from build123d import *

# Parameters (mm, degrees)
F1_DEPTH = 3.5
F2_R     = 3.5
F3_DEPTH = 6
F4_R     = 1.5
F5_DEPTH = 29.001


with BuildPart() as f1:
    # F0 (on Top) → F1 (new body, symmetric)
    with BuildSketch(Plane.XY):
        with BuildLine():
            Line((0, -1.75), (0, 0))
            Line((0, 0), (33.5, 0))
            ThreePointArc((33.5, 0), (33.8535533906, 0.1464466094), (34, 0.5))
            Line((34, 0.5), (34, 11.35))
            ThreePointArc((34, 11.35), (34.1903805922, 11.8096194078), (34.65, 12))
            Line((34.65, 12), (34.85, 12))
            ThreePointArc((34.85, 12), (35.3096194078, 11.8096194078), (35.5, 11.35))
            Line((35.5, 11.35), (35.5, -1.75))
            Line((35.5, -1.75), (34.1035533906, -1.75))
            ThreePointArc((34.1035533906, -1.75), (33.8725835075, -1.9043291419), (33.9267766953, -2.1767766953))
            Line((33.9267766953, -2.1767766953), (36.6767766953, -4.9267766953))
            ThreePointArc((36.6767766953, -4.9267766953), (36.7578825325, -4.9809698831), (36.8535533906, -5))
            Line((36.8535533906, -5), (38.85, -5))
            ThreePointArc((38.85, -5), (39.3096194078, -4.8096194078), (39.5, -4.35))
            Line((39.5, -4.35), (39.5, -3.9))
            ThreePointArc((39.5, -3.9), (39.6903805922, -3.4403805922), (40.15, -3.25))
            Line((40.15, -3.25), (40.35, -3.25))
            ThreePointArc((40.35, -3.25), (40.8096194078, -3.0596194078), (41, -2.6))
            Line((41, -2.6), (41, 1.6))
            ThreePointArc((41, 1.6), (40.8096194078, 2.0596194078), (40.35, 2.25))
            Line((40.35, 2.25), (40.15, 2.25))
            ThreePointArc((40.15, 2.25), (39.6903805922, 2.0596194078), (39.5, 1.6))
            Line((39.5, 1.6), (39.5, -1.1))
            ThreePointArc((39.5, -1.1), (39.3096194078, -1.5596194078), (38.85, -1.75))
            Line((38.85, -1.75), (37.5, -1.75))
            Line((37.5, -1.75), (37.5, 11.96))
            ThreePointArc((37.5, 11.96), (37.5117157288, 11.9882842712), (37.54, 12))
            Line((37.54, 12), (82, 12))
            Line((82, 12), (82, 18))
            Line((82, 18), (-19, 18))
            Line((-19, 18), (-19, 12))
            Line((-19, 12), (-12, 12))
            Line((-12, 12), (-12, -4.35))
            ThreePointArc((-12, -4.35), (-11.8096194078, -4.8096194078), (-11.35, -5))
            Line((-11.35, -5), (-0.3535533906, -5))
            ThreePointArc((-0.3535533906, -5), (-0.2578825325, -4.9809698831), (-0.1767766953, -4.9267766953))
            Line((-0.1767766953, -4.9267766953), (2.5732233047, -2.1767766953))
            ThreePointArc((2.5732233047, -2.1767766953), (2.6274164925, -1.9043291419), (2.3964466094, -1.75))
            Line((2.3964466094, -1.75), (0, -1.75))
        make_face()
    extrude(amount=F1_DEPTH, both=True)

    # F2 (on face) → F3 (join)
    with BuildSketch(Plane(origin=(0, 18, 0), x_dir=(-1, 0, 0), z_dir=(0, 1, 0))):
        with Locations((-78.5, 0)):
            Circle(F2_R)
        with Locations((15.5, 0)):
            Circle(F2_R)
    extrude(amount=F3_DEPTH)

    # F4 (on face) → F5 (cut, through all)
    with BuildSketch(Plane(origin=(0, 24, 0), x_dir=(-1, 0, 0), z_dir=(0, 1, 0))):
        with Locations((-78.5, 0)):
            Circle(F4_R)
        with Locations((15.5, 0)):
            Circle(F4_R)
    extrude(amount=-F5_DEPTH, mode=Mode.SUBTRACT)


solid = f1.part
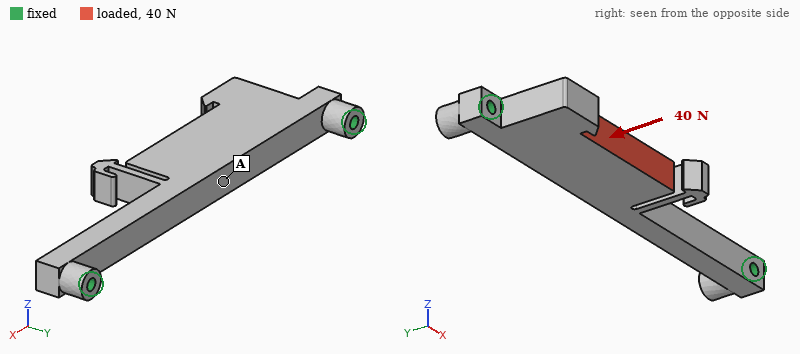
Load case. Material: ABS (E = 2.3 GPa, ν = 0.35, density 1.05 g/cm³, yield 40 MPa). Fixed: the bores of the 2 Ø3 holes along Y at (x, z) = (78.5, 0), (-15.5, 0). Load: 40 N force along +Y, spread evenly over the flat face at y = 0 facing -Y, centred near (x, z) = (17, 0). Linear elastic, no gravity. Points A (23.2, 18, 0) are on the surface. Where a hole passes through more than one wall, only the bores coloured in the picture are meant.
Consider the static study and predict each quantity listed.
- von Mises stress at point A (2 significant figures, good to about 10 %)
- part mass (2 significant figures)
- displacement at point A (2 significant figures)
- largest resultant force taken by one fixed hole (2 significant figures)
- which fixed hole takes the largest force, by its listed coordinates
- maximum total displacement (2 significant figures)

1.1 MPa
9.7 g
0.20 mm
29 N
(-15.5, 0)
0.27 mm
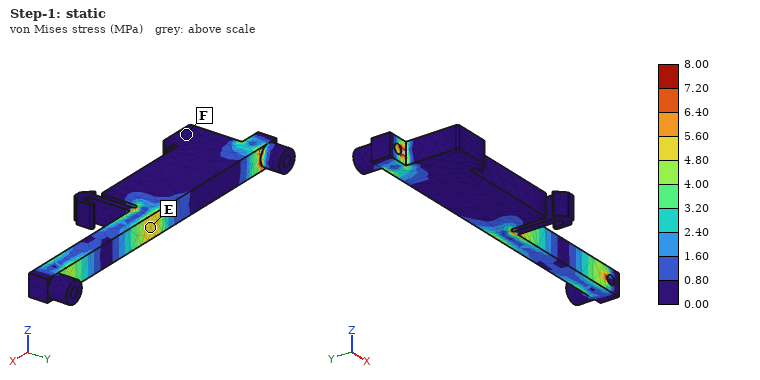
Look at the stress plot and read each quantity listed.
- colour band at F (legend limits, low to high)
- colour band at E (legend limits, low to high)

0.00 to 0.80 MPa
4.80 to 5.60 MPa
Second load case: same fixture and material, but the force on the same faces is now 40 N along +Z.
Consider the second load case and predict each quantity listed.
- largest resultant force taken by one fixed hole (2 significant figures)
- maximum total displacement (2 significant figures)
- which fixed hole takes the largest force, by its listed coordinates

28 N
0.59 mm
(-15.5, 0)
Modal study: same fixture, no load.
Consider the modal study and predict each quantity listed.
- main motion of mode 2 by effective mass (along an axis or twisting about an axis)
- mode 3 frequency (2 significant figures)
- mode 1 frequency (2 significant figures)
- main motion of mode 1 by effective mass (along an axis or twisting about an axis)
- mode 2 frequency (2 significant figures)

along Y
1100 Hz
770 Hz
along Z
840 Hz
